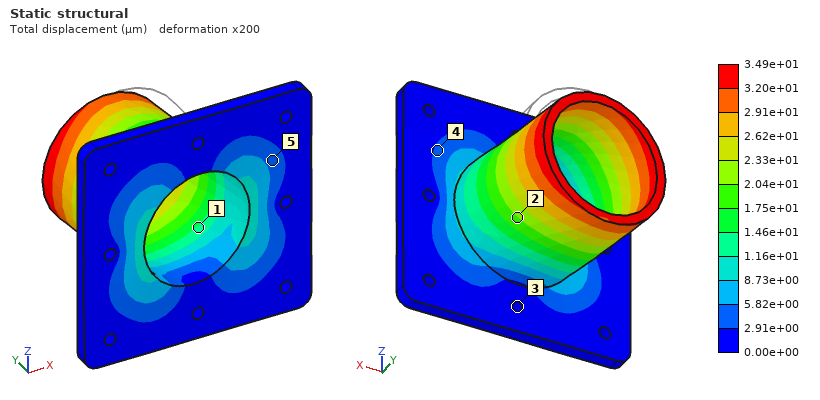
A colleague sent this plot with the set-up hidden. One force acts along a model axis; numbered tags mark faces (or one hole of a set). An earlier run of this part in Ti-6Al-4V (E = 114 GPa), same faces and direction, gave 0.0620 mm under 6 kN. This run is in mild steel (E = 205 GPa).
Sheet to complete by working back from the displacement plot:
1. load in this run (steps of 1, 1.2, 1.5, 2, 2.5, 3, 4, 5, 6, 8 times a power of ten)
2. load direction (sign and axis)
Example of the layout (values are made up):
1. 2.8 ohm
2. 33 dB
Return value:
1. 6 kN
2. -X
